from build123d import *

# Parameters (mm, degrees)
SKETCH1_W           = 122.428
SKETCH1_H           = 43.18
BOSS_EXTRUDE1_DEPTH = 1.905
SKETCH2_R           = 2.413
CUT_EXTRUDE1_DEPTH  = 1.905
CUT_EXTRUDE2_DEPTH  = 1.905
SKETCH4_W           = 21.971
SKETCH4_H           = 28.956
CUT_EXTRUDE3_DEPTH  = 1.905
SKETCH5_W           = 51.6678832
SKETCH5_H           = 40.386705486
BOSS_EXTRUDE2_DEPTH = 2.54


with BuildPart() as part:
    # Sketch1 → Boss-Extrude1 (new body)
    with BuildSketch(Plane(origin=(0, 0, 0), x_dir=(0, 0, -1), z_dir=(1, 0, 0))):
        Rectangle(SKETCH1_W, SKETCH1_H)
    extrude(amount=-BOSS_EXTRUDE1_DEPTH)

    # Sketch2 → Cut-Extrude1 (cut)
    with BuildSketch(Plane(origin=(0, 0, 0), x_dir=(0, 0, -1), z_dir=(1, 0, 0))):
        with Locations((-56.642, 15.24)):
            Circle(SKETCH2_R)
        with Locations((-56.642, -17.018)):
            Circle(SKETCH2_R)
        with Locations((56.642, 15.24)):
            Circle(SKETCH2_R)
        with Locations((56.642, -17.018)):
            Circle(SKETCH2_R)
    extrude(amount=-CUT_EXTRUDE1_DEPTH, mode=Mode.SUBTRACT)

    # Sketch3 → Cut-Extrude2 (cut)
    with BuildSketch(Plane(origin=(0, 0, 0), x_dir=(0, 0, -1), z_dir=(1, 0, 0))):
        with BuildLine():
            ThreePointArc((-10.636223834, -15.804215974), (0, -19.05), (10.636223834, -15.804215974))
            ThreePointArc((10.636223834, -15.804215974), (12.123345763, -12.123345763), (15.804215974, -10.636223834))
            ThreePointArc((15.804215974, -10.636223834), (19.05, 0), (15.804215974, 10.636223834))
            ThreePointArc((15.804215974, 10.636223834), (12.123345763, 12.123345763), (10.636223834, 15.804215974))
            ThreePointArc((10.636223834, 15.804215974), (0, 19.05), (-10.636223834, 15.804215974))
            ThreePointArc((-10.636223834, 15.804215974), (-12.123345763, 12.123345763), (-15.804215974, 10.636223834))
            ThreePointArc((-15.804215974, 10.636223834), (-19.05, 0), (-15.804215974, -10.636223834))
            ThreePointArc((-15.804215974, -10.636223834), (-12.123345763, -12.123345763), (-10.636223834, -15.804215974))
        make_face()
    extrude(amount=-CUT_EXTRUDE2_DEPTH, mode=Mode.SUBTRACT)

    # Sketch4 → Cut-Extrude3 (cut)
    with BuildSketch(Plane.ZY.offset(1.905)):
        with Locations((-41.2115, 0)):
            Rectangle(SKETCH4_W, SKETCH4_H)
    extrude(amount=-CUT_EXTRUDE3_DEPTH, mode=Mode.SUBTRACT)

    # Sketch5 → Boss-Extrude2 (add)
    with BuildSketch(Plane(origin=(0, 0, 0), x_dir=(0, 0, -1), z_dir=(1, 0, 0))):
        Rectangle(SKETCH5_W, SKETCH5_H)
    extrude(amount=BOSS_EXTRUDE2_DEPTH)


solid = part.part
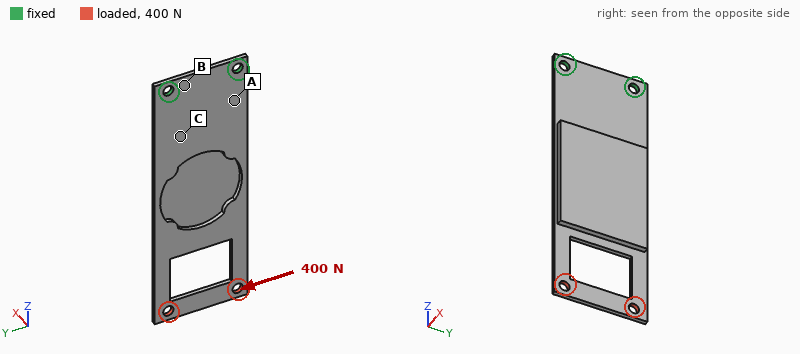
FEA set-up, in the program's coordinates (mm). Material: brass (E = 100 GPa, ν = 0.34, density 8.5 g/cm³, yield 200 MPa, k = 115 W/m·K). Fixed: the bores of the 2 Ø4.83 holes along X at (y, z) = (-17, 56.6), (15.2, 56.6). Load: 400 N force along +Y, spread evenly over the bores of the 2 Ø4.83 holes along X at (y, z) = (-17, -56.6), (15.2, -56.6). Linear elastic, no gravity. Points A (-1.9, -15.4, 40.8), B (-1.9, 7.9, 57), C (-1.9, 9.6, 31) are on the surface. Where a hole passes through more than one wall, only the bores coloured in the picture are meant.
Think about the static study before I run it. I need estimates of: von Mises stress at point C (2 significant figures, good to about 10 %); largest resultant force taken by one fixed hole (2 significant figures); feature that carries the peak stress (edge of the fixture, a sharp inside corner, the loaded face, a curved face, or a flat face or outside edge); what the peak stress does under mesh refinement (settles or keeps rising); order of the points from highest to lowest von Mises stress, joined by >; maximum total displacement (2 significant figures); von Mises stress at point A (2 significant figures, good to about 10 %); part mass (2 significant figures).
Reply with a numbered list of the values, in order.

1. 26 MPa
2. 1.4 kN
3. a sharp inside corner
4. keeps rising
5. A > C > B
6. 0.33 mm
7. 46 MPa
8. 100 g
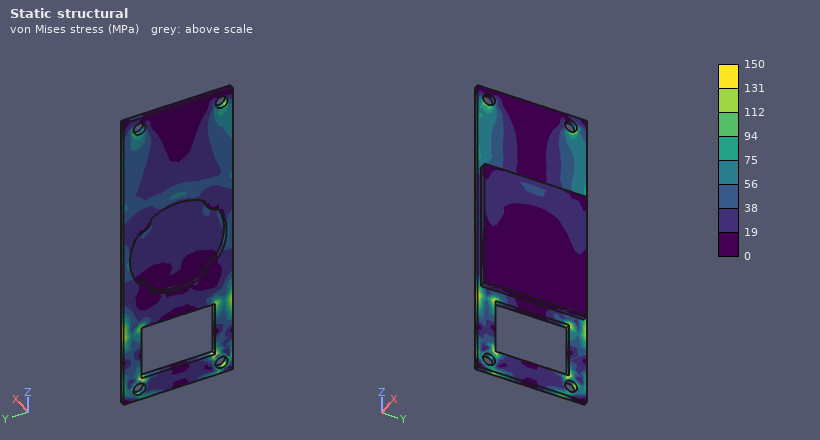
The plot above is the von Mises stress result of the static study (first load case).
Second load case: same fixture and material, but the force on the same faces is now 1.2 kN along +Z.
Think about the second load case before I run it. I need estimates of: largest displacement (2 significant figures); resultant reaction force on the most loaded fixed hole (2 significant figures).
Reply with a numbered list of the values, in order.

1. 0.47 mm
2. 620 N
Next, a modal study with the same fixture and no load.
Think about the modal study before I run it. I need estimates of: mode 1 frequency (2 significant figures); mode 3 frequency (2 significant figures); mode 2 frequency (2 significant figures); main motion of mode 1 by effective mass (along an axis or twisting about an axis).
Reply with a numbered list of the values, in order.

1. 92 Hz
2. 580 Hz
3. 570 Hz
4. along X
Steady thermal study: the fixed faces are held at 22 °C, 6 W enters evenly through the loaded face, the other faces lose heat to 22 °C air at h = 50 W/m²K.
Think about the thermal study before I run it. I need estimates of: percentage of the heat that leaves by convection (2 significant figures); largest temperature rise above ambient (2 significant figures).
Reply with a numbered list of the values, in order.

1. 85 %
2. 48 K
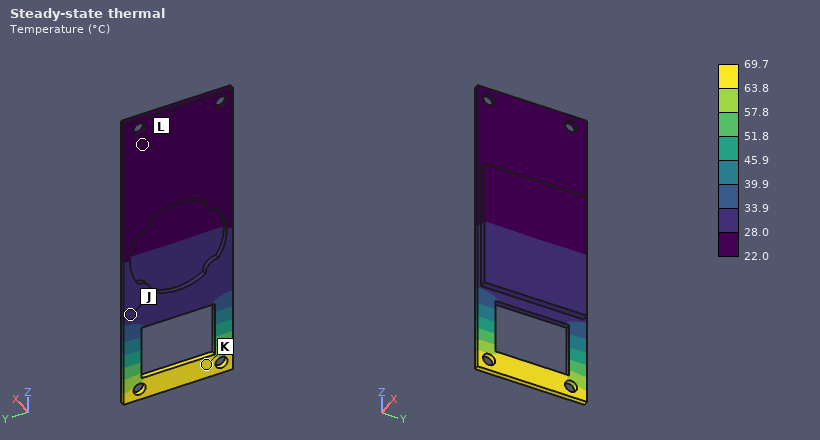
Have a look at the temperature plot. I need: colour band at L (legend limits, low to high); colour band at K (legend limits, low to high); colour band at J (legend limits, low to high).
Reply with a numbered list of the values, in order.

1. 22.0 to 28.0 °C
2. 63.8 to 69.7 °C
3. 28.0 to 33.9 °C
